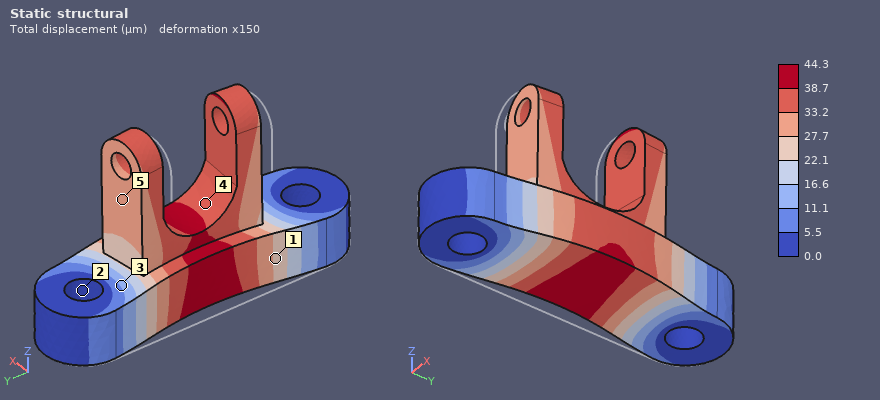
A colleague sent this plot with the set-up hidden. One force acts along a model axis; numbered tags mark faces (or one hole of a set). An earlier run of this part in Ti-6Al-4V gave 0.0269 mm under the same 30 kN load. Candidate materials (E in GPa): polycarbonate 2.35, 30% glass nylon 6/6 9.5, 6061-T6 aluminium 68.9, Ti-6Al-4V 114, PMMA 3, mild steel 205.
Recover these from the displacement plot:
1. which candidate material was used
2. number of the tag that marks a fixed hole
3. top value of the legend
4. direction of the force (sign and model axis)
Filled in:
6061-T6 aluminium
2
44.3 µm
+X
